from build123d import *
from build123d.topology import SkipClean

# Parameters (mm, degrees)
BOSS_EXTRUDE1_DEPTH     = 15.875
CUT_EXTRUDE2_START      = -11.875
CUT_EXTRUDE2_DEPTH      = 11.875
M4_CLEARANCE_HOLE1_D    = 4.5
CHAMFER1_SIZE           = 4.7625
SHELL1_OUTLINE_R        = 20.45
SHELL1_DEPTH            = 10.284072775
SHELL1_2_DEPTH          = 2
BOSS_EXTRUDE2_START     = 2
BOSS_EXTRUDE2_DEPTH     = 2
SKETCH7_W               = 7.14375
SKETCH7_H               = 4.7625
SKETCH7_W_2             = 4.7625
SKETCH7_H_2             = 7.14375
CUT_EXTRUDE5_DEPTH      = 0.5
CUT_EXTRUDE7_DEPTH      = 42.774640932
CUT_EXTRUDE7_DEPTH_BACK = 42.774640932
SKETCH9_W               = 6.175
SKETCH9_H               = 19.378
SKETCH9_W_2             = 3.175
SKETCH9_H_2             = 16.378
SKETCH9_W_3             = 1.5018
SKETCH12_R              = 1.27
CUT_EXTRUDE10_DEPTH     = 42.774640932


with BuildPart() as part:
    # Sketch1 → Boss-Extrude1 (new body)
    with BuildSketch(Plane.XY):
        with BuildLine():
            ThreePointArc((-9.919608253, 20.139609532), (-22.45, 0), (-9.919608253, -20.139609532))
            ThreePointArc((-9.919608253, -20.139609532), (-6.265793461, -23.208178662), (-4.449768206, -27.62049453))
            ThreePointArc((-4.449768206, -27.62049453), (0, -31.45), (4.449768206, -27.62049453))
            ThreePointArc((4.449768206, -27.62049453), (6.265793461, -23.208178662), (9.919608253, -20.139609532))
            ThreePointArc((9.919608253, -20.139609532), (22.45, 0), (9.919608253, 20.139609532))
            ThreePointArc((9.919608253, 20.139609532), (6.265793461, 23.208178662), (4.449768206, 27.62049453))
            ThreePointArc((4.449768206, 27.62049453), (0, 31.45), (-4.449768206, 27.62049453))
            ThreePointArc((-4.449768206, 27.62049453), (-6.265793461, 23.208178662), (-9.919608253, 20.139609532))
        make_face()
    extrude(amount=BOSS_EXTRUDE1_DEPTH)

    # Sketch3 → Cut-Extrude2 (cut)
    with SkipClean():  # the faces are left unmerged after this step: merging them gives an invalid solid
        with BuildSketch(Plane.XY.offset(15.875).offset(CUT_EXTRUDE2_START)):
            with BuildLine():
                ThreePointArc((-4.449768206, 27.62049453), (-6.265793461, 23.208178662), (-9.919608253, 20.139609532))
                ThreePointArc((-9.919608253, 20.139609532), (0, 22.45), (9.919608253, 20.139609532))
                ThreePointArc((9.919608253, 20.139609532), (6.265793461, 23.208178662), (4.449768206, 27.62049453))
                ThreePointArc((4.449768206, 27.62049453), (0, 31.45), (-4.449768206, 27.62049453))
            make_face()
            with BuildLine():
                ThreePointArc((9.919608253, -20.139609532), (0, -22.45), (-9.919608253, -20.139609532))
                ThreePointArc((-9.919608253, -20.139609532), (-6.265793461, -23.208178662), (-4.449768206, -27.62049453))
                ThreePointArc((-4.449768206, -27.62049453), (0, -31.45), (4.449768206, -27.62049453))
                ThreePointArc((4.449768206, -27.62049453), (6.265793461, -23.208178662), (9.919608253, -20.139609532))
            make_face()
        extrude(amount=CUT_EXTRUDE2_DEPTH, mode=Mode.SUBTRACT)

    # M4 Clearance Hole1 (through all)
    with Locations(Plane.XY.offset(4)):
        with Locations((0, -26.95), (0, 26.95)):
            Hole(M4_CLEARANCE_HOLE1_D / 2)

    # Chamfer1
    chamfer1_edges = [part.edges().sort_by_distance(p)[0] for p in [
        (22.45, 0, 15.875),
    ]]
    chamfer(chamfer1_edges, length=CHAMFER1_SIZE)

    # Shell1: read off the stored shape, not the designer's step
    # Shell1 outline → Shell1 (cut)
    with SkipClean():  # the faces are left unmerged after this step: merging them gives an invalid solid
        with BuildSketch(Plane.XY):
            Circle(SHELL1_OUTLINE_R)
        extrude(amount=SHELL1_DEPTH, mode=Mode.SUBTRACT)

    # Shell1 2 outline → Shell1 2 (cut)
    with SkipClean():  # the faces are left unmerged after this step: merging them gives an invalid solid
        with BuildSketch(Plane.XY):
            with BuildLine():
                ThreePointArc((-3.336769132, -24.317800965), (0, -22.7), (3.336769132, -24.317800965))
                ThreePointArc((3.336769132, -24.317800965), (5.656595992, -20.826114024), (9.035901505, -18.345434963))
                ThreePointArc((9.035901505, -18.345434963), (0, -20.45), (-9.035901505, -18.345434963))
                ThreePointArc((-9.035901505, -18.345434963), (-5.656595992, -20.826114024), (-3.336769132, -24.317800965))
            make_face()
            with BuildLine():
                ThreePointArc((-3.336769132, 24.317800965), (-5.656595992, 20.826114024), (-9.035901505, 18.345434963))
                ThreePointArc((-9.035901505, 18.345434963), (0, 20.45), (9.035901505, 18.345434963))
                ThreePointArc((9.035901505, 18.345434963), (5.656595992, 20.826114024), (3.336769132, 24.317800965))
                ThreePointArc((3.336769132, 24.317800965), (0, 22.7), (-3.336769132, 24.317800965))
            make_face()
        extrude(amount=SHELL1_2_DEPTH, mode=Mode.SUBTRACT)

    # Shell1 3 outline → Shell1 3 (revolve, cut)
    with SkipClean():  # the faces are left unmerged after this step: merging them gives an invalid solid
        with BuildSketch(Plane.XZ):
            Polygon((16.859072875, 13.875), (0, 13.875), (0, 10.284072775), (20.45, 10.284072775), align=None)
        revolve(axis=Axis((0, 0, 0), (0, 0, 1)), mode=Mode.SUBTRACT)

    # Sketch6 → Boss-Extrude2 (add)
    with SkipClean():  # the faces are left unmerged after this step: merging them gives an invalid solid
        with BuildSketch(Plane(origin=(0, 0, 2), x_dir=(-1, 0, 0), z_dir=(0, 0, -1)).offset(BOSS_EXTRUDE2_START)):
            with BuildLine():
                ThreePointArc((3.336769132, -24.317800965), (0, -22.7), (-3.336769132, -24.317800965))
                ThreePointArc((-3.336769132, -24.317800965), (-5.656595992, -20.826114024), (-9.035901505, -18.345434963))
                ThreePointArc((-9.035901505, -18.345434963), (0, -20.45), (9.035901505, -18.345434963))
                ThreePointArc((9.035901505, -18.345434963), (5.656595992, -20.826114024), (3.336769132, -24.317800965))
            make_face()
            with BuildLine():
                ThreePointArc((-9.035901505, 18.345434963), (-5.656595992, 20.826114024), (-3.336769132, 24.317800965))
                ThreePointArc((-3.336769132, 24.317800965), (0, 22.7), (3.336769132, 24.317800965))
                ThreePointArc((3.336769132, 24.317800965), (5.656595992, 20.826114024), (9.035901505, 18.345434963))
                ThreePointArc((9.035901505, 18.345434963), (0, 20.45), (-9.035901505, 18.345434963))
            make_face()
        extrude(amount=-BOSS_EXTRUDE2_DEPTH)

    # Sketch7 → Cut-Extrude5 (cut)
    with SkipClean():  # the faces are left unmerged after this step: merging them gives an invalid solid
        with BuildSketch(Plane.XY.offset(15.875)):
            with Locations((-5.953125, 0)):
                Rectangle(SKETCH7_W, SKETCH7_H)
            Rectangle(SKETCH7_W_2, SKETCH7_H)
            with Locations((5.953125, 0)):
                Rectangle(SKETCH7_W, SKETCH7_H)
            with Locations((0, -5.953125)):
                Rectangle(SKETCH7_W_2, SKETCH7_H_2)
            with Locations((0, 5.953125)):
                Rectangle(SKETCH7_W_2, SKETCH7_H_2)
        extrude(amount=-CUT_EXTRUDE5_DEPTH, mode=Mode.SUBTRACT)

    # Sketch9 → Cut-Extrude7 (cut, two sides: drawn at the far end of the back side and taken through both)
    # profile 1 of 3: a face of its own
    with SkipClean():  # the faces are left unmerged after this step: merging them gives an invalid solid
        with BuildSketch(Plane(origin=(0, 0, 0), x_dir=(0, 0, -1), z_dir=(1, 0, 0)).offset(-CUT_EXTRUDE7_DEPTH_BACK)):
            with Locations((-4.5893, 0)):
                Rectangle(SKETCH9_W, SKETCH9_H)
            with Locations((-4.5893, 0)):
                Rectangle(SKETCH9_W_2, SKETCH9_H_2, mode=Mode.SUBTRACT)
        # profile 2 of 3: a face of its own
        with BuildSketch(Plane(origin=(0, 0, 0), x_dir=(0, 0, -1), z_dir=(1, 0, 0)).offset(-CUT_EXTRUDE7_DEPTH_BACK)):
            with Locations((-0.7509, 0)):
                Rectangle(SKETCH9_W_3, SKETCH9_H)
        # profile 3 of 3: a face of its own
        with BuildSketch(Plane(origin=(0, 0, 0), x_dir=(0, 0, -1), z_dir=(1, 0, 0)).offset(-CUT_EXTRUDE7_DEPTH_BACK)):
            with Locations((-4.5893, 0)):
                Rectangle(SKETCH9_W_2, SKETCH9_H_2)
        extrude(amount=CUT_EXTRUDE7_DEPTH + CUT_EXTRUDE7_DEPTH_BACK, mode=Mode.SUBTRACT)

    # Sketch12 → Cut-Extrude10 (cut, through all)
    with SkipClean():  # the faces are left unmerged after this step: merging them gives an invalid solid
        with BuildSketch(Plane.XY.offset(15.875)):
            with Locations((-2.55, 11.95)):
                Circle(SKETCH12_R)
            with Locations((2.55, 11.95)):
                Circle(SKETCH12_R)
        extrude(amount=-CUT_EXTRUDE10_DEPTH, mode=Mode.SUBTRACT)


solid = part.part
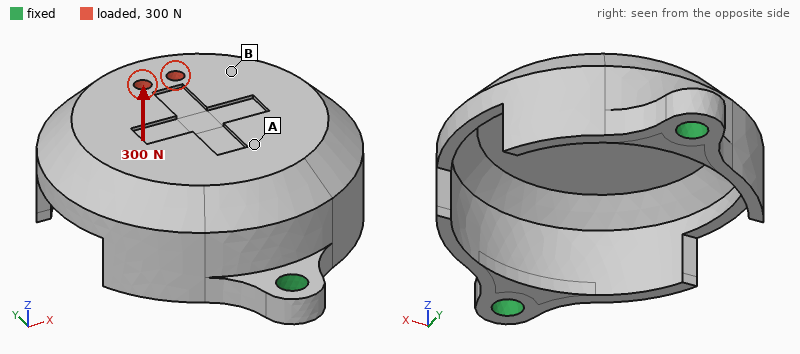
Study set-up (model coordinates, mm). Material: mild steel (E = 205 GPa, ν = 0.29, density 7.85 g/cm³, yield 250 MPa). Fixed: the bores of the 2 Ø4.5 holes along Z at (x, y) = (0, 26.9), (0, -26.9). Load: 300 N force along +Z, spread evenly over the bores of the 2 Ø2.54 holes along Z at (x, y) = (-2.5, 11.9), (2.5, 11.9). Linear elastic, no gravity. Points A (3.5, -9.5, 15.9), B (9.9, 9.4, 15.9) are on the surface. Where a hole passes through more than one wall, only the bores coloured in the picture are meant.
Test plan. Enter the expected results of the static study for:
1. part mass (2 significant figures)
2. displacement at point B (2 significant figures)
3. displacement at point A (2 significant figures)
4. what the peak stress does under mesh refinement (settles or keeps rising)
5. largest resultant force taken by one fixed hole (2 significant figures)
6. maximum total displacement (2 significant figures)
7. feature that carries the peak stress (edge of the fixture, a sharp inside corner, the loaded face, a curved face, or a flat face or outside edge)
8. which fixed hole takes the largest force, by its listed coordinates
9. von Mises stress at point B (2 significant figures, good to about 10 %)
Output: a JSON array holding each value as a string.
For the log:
["48 g", "5.0 µm", "2.0 µm", "keeps rising", "250 N", "11 µm", "a sharp inside corner", "(0, 26.9)", "21 MPa"]
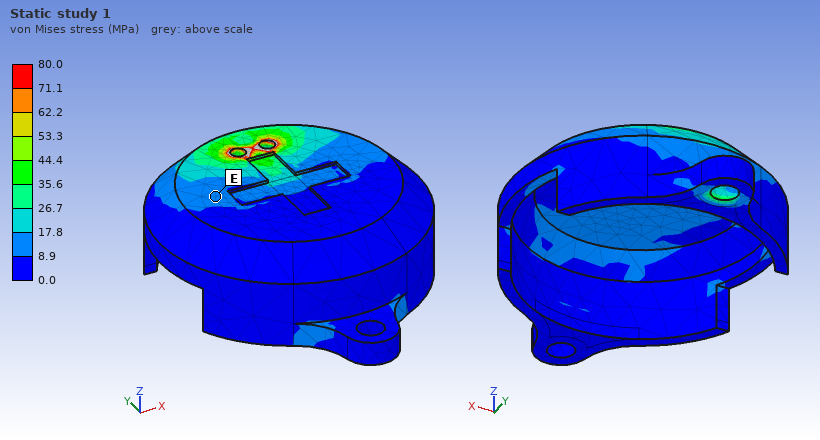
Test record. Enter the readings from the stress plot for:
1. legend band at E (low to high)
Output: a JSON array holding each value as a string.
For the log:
["8.9 to 17.8 MPa"]
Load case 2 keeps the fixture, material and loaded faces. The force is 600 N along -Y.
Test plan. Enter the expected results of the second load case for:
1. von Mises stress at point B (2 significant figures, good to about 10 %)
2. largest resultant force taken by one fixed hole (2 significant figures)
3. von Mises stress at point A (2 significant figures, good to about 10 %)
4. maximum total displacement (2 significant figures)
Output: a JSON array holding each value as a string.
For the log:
["10 MPa", "330 N", "7.7 MPa", "14 µm"]
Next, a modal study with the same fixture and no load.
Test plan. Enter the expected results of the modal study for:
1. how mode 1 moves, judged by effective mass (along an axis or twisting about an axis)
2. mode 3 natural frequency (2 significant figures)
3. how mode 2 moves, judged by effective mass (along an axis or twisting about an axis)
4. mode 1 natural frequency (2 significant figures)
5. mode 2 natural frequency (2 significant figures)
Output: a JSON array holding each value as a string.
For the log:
["along X", "7500 Hz", "along Y", "4000 Hz", "6400 Hz"]
